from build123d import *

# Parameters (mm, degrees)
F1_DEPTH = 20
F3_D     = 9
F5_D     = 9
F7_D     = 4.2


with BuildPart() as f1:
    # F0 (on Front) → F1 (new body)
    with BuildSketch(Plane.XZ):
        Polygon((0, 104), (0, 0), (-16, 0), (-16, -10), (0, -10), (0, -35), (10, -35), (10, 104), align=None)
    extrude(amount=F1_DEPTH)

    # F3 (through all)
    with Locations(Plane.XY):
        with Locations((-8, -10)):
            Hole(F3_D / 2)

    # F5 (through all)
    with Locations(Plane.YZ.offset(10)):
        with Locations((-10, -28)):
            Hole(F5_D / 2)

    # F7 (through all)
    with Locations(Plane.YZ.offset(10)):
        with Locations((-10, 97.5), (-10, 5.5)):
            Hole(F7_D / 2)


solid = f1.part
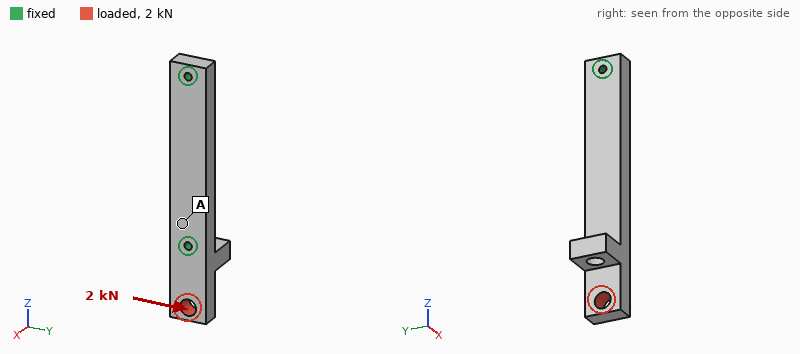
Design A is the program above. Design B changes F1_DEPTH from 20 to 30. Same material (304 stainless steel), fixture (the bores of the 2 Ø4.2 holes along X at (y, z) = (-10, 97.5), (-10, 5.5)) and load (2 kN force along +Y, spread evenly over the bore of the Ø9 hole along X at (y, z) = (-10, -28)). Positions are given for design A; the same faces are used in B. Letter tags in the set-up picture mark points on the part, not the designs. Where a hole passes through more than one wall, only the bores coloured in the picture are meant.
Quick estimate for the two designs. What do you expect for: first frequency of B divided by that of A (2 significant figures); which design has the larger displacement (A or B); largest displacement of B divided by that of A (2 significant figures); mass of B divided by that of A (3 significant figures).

0.85
A
0.42
1.53
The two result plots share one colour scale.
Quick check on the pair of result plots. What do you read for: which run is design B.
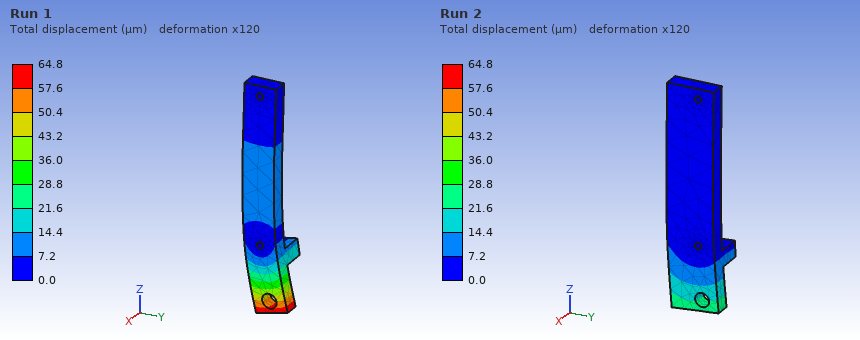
Run 2
